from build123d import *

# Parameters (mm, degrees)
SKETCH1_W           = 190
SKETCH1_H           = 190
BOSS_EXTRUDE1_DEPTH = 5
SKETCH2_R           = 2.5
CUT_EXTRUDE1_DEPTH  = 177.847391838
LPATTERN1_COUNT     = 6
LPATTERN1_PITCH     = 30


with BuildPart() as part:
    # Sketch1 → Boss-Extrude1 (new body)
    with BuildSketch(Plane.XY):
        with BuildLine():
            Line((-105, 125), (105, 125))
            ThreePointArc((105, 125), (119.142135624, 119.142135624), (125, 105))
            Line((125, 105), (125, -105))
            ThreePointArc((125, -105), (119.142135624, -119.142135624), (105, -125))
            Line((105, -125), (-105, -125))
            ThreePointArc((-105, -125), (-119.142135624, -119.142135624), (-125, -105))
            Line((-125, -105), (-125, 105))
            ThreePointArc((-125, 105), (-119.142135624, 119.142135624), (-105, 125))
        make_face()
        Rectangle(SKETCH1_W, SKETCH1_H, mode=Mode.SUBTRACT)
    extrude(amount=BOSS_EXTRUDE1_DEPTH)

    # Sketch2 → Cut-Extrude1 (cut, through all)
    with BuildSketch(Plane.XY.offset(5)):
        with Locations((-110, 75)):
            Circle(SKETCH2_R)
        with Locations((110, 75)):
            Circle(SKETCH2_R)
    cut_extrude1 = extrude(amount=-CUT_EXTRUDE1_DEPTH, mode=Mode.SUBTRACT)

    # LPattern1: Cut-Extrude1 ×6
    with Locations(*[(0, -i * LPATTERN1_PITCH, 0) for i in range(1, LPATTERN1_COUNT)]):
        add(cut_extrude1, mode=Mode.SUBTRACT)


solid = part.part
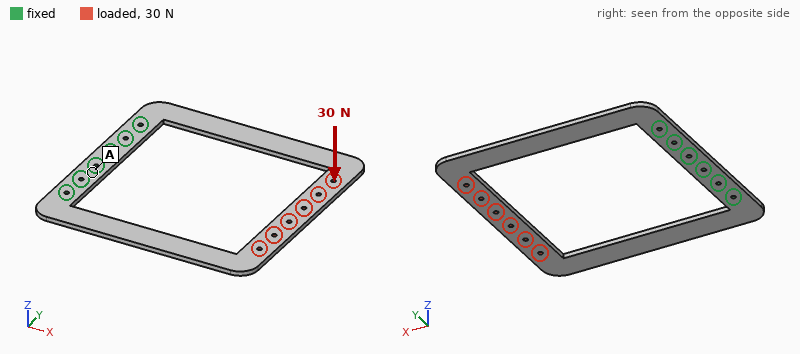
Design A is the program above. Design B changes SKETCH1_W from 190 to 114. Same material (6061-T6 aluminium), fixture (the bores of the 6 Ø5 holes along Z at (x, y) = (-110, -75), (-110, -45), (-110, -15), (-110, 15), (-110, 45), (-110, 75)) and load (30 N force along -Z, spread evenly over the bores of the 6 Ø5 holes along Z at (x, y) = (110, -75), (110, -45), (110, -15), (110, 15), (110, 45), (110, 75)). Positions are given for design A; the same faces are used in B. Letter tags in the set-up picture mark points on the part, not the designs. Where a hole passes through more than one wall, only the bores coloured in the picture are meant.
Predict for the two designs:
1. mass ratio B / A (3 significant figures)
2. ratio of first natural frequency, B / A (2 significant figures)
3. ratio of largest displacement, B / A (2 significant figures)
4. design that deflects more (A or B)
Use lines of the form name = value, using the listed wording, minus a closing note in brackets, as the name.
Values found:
mass ratio B / A = 1.56
ratio of first natural frequency, B / A = 1.1
ratio of largest displacement, B / A = 0.64
design that deflects more = A
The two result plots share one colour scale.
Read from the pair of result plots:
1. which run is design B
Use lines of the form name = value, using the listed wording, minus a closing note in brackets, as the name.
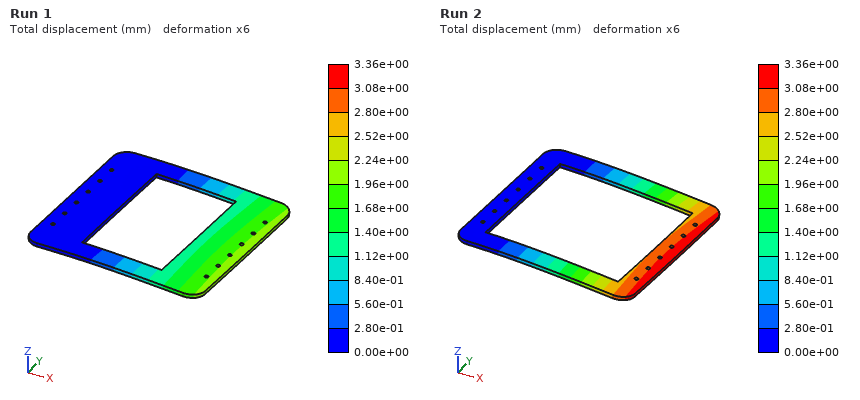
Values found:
which run is design B = Run 1
